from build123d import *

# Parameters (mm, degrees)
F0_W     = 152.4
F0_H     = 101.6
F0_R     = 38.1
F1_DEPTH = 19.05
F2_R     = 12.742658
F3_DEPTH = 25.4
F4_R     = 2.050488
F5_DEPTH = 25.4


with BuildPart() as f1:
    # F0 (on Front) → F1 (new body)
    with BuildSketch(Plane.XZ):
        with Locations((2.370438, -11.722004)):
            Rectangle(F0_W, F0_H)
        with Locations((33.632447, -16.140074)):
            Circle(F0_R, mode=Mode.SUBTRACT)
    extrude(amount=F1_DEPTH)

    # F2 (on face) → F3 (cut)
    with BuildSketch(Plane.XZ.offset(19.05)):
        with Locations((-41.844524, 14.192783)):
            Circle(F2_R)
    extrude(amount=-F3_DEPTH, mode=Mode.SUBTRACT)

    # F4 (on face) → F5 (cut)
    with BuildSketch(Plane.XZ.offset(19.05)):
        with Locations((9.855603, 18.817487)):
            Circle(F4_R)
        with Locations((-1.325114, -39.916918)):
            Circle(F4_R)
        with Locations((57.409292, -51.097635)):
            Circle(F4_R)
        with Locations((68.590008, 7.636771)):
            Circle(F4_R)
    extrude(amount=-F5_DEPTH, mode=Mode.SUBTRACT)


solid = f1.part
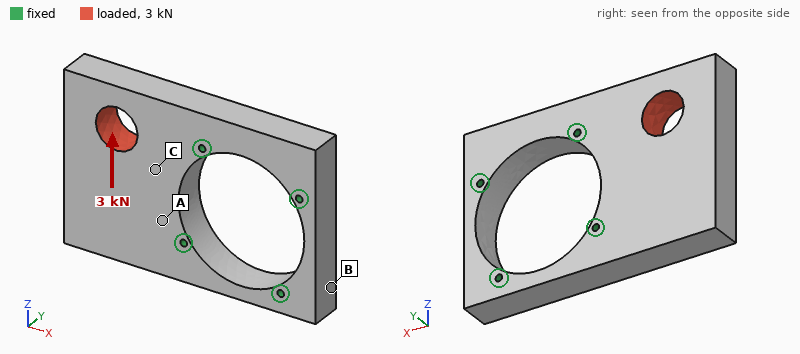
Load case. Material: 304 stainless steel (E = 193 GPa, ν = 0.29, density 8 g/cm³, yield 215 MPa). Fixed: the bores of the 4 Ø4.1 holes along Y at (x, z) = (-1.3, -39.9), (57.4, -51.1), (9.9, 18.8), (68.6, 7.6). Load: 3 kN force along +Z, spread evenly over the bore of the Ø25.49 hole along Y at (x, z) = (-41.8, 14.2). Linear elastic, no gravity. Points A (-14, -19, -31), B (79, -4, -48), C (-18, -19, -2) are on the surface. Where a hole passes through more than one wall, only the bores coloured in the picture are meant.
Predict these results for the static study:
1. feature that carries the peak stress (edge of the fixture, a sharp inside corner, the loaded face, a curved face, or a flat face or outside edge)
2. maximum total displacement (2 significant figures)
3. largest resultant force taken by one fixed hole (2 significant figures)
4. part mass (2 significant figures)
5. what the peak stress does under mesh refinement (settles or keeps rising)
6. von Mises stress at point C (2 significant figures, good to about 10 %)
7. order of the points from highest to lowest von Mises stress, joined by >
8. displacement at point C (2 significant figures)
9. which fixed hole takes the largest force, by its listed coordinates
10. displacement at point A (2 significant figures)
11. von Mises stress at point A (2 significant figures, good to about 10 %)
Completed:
edge of the fixture
3.7 µm
2.4 kN
1.6 kg
keeps rising
6.1 MPa
C > A > B
1.4 µm
(-1.3, -39.9)
0.92 µm
4.3 MPa
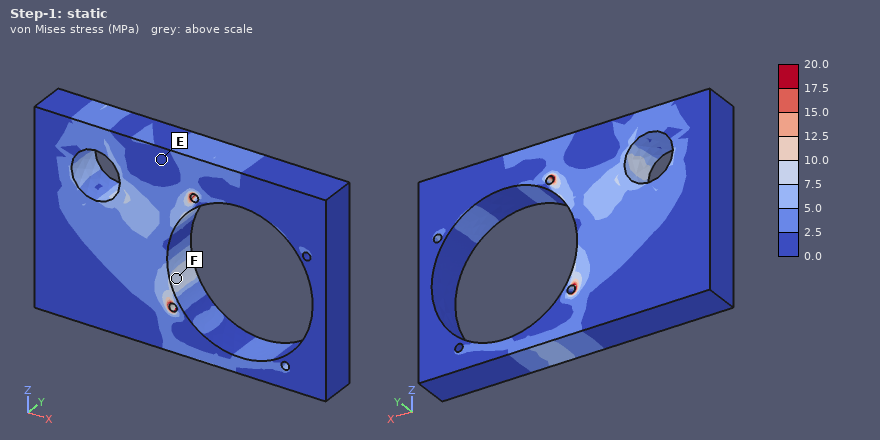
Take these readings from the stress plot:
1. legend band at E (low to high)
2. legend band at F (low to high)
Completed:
0.0 to 2.5 MPa
7.5 to 10.0 MPa
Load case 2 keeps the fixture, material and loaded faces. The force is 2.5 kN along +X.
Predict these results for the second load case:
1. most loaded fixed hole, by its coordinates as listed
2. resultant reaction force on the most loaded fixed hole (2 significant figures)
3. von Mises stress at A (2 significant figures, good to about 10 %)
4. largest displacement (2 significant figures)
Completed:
(9.9, 18.8)
2.0 kN
1.4 MPa
1.7 µm
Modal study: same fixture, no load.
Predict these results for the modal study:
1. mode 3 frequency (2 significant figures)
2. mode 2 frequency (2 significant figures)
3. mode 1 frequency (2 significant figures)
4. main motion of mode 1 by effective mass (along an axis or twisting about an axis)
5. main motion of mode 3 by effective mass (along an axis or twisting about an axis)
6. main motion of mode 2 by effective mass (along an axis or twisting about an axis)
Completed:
5400 Hz
3800 Hz
1800 Hz
along Y
along Z
twisting about X
